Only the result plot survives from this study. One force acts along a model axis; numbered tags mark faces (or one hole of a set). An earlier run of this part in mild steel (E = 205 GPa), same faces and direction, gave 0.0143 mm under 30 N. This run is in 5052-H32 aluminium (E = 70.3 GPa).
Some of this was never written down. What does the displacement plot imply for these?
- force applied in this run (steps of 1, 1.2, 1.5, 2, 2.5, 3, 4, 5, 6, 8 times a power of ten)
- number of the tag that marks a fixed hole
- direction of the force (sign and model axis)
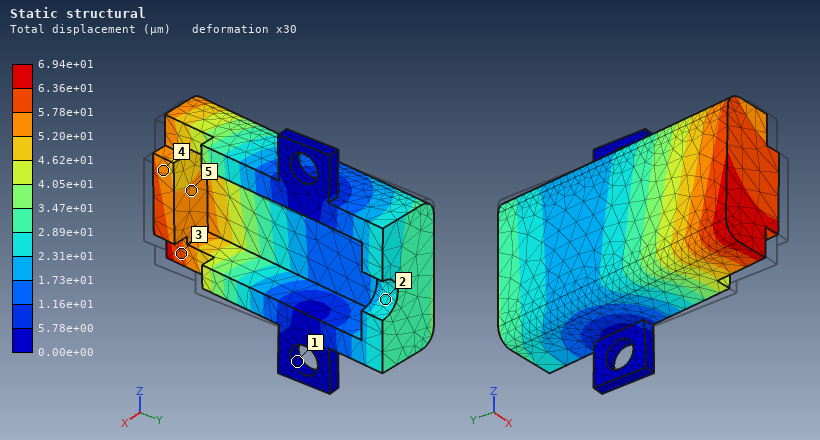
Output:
50 N
1
-X
